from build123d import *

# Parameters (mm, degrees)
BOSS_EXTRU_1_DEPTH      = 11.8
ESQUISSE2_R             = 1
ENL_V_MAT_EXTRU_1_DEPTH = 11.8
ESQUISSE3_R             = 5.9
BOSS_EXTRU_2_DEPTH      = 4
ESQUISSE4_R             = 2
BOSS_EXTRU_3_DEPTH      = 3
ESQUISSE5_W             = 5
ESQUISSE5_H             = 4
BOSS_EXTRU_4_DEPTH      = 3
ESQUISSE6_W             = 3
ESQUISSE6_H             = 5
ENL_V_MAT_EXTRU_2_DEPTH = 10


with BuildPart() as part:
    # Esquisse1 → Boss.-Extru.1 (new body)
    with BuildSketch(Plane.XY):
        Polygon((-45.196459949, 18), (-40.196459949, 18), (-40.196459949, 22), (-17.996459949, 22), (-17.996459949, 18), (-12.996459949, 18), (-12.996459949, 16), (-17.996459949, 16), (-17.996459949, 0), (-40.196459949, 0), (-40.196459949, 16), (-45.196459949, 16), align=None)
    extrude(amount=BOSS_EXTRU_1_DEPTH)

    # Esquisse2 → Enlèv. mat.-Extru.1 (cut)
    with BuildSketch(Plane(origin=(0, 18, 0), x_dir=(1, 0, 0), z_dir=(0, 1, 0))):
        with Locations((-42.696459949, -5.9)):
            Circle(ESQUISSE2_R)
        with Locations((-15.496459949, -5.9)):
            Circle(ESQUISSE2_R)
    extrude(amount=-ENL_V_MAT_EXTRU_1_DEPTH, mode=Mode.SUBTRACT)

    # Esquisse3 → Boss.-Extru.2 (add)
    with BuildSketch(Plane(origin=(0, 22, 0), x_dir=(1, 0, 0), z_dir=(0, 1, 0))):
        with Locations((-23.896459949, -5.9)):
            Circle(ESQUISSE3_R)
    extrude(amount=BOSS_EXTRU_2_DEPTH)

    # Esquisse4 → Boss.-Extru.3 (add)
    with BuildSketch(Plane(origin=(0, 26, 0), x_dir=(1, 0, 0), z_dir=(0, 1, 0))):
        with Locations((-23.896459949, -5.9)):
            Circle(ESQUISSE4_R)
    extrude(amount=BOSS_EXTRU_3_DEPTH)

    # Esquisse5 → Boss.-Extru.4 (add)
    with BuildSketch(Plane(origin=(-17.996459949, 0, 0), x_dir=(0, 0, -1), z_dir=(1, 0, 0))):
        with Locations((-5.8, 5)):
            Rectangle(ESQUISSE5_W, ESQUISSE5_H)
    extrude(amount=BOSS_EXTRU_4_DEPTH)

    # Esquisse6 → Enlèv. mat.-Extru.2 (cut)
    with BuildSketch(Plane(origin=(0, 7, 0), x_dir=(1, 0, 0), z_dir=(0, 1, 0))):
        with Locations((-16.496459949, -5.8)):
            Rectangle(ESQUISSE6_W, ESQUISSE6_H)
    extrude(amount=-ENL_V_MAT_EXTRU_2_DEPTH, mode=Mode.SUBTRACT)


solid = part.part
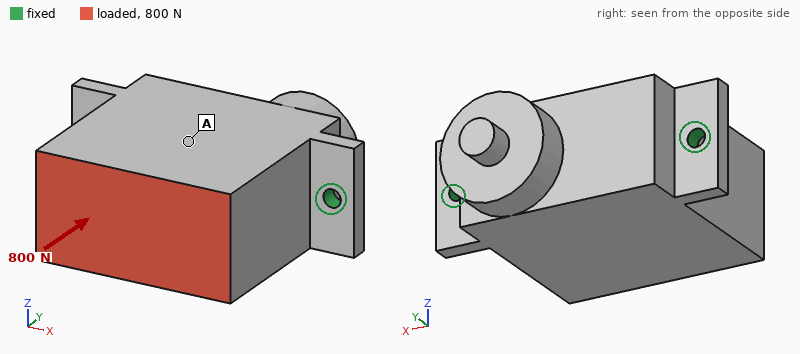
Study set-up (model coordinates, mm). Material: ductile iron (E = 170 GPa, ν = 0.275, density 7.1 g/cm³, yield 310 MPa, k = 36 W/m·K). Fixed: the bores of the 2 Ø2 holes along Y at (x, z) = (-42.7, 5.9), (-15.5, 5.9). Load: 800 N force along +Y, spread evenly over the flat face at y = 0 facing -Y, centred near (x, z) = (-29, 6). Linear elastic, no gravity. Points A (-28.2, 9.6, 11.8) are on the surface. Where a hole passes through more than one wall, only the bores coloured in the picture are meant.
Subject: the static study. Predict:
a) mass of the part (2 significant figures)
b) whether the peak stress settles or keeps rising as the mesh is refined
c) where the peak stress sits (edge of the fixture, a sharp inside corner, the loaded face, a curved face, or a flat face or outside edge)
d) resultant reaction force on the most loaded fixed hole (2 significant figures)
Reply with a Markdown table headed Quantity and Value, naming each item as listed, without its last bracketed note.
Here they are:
| Quantity | Value |
|---|---|
| mass of the part | 46 g |
| whether the peak stress settles or keeps rising as the mesh is refined | keeps rising |
| where the peak stress sits | edge of the fixture |
| resultant reaction force on the most loaded fixed hole | 400 N |
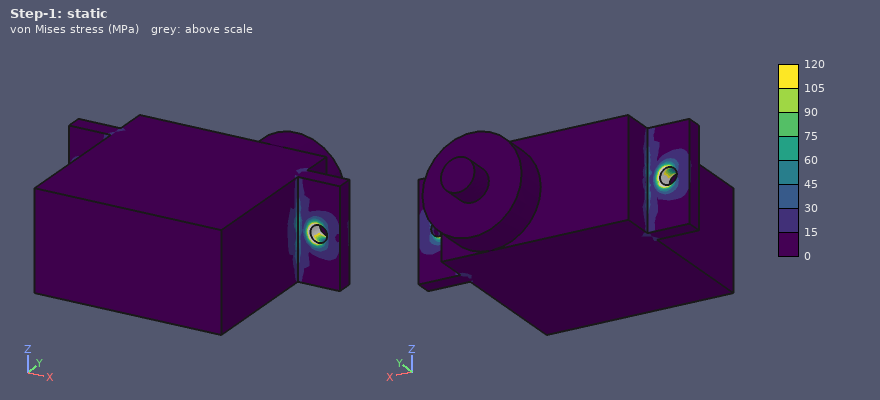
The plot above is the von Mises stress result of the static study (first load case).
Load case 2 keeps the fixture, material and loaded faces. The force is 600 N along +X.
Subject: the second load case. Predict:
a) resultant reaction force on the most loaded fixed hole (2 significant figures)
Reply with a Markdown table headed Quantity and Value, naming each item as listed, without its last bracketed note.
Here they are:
| Quantity | Value |
|---|---|
| resultant reaction force on the most loaded fixed hole | 510 N |
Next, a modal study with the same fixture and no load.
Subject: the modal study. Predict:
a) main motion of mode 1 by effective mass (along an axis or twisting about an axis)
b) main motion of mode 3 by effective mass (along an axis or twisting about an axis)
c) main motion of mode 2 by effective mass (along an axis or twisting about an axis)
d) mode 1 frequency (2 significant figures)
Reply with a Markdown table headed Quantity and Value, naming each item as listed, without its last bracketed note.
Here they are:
| Quantity | Value |
|---|---|
| main motion of mode 1 by effective mass | along Z |
| main motion of mode 3 by effective mass | along X |
| main motion of mode 2 by effective mass | along Y |
| mode 1 frequency | 3100 Hz |
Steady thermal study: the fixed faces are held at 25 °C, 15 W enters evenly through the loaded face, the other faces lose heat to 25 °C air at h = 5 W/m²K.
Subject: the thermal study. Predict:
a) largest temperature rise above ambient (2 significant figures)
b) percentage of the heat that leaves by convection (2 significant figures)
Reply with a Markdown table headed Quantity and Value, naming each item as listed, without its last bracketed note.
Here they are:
| Quantity | Value |
|---|---|
| largest temperature rise above ambient | 69 K |
| percentage of the heat that leaves by convection | 3.3 % |
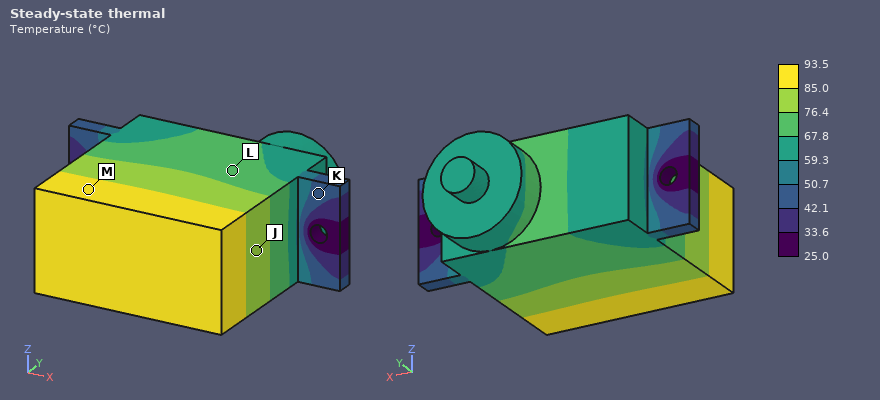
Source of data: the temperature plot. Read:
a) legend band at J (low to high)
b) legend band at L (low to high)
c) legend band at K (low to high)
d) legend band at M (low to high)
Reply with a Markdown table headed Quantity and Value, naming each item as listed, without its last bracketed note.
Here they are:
| Quantity | Value |
|---|---|
| legend band at J | 76.4 to 85.0 °C |
| legend band at L | 67.8 to 76.4 °C |
| legend band at K | 42.1 to 50.7 °C |
| legend band at M | 85.0 to 93.5 °C |
